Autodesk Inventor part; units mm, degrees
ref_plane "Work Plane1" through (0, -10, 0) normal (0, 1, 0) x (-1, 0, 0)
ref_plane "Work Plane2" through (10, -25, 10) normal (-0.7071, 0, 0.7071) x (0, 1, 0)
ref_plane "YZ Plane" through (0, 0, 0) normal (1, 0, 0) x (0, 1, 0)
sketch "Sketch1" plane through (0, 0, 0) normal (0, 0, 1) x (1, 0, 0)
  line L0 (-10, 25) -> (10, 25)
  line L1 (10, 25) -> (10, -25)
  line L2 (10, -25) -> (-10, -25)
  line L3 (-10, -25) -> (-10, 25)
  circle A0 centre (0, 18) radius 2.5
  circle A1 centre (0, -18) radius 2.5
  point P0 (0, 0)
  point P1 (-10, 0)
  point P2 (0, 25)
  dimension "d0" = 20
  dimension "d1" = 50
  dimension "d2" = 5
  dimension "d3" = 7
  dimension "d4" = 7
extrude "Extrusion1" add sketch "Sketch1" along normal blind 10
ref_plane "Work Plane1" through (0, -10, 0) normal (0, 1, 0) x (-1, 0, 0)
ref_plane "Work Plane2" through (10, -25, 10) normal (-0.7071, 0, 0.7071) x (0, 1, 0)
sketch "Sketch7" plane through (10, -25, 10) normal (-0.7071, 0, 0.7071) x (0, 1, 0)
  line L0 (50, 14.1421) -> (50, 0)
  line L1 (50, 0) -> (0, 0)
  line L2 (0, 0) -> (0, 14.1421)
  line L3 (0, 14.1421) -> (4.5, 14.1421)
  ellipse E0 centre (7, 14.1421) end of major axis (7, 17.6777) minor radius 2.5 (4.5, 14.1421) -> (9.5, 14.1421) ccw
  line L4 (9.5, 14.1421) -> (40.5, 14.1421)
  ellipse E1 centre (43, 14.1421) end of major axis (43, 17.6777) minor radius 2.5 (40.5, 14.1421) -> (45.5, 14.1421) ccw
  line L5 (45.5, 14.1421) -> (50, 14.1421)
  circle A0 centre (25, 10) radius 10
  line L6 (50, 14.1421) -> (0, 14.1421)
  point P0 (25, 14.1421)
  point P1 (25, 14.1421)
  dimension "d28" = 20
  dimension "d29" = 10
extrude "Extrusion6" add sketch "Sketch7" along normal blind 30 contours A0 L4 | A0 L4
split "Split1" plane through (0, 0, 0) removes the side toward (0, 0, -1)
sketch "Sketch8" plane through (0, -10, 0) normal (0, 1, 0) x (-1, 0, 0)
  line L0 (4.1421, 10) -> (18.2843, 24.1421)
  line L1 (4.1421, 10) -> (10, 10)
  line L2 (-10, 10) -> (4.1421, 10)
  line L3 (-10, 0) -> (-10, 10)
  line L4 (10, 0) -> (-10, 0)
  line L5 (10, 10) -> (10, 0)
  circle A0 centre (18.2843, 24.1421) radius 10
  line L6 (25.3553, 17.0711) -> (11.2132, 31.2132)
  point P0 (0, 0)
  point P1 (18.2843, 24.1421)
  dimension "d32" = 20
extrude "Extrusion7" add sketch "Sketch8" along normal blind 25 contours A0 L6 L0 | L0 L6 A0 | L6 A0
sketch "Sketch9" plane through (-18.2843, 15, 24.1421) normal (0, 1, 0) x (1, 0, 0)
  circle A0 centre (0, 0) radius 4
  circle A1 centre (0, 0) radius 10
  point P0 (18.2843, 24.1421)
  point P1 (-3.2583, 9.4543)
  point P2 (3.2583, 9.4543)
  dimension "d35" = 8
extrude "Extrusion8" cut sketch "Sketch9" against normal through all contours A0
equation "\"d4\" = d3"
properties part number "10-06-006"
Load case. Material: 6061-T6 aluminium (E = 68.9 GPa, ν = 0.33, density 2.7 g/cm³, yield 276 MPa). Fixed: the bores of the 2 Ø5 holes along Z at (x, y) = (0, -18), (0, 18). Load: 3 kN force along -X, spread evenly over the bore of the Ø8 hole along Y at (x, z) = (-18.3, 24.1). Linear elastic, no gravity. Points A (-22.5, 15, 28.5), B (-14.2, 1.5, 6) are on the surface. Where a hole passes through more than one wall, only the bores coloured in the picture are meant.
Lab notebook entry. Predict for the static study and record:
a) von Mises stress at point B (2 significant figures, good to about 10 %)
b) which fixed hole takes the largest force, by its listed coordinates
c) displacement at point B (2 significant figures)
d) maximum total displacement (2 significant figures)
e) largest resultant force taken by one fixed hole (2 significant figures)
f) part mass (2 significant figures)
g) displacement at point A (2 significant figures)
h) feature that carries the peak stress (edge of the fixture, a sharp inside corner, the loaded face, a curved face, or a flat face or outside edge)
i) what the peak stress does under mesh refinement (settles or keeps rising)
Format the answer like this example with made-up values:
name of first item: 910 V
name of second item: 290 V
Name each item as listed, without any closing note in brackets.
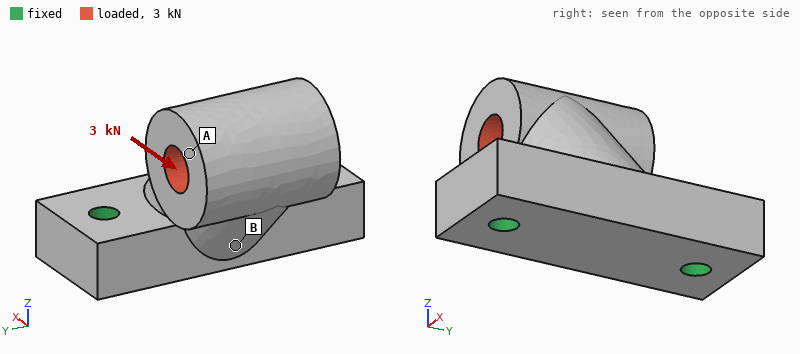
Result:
von Mises stress at point B: 35 MPa
which fixed hole takes the largest force, by its listed coordinates: (0, 18)
displacement at point B: 0.045 mm
maximum total displacement: 0.14 mm
largest resultant force taken by one fixed hole: 1.7 kN
part mass: 55 g
displacement at point A: 0.13 mm
feature that carries the peak stress: edge of the fixture
what the peak stress does under mesh refinement: keeps rising
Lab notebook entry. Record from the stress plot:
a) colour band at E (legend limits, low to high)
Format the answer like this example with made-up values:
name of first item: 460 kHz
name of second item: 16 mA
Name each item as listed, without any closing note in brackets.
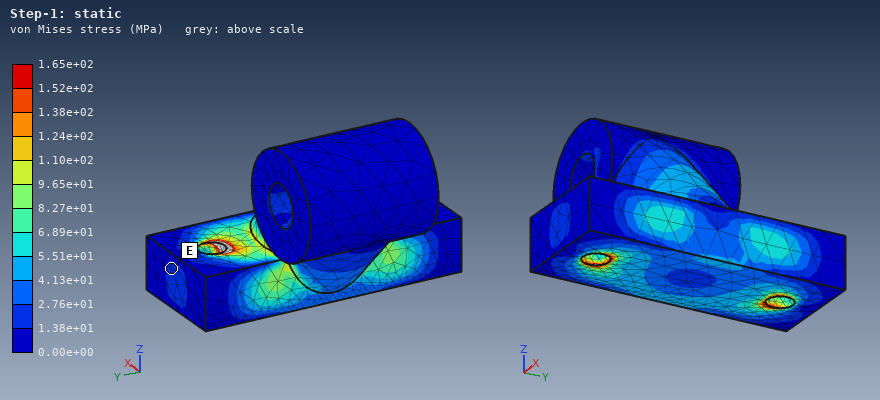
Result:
colour band at E: 1.38e+01 to 2.76e+01 MPa
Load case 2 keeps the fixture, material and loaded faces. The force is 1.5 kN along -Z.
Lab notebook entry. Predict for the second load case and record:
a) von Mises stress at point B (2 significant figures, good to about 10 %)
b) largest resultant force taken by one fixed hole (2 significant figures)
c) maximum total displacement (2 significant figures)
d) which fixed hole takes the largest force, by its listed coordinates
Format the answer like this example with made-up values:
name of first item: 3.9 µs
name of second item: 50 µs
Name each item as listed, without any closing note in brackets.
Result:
von Mises stress at point B: 19 MPa
largest resultant force taken by one fixed hole: 920 N
maximum total displacement: 68 µm
which fixed hole takes the largest force, by its listed coordinates: (0, 18)
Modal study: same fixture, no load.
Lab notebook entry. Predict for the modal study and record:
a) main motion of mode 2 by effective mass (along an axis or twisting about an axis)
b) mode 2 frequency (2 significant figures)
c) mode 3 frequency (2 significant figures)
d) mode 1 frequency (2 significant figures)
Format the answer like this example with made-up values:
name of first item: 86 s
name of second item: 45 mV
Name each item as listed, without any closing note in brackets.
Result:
main motion of mode 2 by effective mass: along Y
mode 2 frequency: 9000 Hz
mode 3 frequency: 17 kHz
mode 1 frequency: 5000 Hz
